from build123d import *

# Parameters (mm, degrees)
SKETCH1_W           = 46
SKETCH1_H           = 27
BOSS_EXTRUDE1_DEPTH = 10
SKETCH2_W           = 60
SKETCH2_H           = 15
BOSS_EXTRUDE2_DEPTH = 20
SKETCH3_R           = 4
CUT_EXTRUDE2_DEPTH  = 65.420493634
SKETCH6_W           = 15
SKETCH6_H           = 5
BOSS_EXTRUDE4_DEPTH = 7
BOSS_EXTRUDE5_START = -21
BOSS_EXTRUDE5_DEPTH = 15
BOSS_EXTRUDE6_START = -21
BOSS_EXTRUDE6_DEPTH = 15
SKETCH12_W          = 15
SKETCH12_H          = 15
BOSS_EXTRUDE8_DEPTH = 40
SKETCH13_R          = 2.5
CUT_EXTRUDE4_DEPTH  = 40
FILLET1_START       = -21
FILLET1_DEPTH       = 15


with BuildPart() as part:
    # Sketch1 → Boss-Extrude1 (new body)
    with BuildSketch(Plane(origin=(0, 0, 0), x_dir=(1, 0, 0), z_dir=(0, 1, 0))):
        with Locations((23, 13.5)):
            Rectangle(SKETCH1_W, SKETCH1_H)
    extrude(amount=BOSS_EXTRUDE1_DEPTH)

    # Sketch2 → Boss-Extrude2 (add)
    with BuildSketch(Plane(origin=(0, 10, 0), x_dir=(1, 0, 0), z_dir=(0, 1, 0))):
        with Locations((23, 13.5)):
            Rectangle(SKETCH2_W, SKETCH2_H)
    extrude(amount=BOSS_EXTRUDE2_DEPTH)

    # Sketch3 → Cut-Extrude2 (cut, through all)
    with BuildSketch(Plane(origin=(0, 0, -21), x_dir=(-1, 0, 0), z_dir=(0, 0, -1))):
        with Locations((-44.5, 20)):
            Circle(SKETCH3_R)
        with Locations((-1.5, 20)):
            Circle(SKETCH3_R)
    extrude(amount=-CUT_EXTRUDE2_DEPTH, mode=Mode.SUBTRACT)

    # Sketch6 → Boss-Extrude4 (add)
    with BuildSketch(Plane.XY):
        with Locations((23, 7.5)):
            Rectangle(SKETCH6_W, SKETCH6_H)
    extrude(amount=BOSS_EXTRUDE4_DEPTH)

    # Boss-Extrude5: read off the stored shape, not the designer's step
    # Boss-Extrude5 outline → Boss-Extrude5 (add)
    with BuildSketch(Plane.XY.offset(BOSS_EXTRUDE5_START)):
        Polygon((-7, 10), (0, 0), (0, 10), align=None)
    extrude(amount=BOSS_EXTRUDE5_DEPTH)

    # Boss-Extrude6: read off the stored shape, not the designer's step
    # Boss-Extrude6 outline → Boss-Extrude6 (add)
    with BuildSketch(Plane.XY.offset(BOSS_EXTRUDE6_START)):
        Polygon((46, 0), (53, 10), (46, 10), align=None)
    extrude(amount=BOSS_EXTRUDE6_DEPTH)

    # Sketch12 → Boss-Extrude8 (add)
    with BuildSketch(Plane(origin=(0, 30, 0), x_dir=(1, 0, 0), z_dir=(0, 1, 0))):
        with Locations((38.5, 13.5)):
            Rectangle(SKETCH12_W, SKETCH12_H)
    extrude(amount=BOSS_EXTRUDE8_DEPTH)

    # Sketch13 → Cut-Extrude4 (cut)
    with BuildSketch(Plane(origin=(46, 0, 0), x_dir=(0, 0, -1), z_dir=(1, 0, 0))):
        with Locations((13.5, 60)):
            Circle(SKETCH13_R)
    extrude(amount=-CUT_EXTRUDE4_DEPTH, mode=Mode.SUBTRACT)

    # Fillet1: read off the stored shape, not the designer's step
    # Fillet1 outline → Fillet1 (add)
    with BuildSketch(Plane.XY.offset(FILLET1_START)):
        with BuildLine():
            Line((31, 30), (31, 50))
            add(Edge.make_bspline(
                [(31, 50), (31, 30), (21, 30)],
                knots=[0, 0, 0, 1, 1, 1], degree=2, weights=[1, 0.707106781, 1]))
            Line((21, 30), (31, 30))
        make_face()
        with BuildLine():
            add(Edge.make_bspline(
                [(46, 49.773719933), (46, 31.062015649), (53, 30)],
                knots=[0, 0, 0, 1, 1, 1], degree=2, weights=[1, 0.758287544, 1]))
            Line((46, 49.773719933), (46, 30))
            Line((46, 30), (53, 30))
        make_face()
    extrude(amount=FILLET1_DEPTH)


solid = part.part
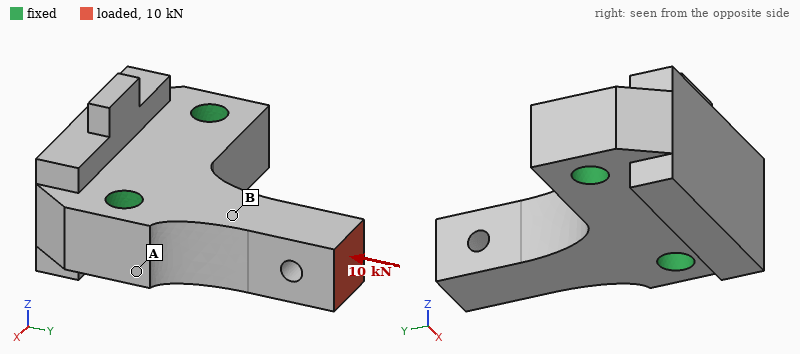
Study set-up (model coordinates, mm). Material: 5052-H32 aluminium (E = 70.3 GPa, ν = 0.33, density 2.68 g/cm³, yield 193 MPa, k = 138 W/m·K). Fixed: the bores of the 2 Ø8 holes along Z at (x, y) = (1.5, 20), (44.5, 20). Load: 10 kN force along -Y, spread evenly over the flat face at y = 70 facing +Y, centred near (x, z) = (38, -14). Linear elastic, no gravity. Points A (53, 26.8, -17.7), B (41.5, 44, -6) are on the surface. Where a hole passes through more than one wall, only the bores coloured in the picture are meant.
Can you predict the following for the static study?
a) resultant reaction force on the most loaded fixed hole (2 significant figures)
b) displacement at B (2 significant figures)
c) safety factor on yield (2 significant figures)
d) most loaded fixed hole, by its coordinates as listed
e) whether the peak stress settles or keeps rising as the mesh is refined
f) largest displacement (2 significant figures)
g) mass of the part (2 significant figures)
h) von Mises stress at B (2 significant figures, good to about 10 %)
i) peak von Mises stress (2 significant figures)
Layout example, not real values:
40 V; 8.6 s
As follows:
8.6 kN; 12 µm; 1.3; (44.5, 20); settles; 33 µm; 110 g; 41 MPa; 150 MPa
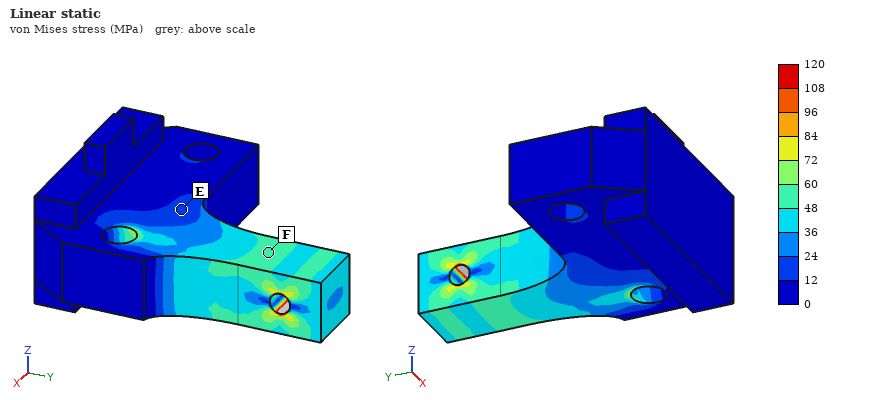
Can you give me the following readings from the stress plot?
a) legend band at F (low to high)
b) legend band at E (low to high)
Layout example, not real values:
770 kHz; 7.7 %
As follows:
48 to 60 MPa; 12 to 24 MPa
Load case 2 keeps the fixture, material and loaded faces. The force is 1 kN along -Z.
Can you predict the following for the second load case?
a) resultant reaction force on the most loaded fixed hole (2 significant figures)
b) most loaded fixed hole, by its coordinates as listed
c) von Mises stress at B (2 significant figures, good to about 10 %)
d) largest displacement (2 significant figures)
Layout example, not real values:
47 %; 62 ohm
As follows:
1.1 kN; (44.5, 20); 43 MPa; 0.11 mm
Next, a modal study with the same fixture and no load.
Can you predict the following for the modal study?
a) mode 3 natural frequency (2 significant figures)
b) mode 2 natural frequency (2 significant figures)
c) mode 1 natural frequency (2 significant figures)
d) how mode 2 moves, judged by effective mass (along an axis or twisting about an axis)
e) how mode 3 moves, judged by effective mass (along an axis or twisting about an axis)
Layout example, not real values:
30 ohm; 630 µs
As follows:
15 kHz; 8100 Hz; 5800 Hz; along X; along Z
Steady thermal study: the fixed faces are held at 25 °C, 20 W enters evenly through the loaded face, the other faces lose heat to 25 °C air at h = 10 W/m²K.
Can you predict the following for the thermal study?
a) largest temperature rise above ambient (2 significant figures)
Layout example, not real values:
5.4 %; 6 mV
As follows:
29 K
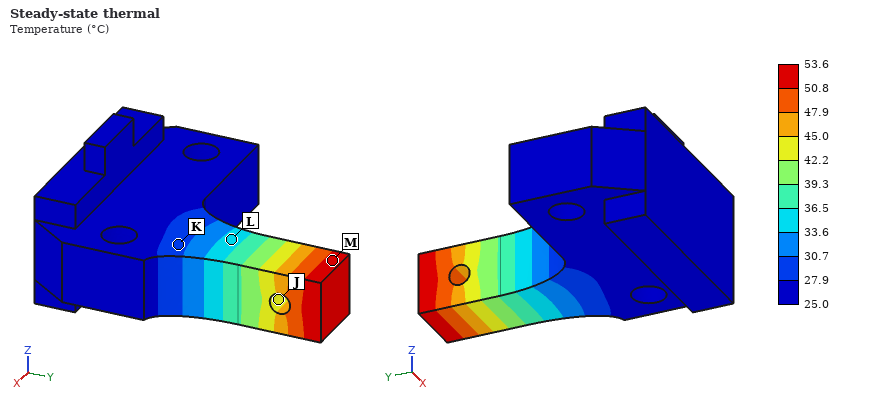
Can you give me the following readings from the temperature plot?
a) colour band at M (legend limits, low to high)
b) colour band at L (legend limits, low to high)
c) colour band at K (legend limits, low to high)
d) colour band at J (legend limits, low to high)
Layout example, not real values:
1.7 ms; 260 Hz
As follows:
50.8 to 53.6 °C; 33.6 to 36.5 °C; 27.9 to 30.7 °C; 42.2 to 45.0 °C
